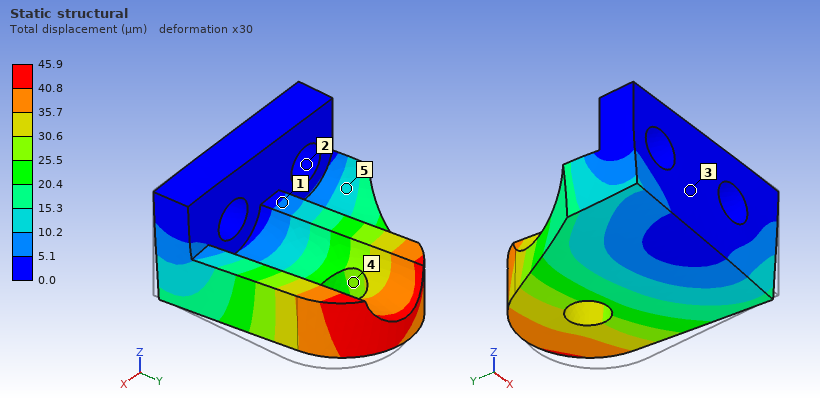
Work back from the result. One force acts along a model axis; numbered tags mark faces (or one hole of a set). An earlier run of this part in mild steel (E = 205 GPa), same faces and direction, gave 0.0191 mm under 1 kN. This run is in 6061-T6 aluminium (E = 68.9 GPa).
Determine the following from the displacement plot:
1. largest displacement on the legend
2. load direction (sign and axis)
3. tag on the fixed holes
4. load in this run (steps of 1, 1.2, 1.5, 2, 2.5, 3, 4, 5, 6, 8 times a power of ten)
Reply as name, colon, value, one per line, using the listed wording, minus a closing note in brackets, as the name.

largest displacement on the legend: 45.9 µm
load direction: -X
tag on the fixed holes: 2
load in this run: 800 N
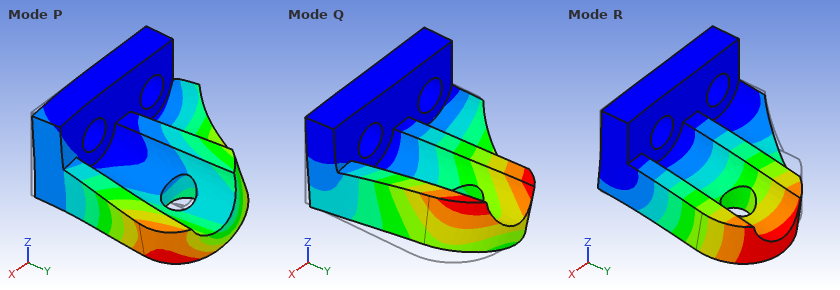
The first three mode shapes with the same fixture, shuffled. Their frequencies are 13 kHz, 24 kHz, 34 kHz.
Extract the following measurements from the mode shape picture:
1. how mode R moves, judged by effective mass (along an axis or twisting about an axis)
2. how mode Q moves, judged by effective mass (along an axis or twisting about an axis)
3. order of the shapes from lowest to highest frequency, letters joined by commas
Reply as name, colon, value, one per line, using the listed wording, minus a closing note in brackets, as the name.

how mode R moves, judged by effective mass: along Z
how mode Q moves, judged by effective mass: along X
order of the shapes from lowest to highest frequency, letters joined by commas: R, Q, P
